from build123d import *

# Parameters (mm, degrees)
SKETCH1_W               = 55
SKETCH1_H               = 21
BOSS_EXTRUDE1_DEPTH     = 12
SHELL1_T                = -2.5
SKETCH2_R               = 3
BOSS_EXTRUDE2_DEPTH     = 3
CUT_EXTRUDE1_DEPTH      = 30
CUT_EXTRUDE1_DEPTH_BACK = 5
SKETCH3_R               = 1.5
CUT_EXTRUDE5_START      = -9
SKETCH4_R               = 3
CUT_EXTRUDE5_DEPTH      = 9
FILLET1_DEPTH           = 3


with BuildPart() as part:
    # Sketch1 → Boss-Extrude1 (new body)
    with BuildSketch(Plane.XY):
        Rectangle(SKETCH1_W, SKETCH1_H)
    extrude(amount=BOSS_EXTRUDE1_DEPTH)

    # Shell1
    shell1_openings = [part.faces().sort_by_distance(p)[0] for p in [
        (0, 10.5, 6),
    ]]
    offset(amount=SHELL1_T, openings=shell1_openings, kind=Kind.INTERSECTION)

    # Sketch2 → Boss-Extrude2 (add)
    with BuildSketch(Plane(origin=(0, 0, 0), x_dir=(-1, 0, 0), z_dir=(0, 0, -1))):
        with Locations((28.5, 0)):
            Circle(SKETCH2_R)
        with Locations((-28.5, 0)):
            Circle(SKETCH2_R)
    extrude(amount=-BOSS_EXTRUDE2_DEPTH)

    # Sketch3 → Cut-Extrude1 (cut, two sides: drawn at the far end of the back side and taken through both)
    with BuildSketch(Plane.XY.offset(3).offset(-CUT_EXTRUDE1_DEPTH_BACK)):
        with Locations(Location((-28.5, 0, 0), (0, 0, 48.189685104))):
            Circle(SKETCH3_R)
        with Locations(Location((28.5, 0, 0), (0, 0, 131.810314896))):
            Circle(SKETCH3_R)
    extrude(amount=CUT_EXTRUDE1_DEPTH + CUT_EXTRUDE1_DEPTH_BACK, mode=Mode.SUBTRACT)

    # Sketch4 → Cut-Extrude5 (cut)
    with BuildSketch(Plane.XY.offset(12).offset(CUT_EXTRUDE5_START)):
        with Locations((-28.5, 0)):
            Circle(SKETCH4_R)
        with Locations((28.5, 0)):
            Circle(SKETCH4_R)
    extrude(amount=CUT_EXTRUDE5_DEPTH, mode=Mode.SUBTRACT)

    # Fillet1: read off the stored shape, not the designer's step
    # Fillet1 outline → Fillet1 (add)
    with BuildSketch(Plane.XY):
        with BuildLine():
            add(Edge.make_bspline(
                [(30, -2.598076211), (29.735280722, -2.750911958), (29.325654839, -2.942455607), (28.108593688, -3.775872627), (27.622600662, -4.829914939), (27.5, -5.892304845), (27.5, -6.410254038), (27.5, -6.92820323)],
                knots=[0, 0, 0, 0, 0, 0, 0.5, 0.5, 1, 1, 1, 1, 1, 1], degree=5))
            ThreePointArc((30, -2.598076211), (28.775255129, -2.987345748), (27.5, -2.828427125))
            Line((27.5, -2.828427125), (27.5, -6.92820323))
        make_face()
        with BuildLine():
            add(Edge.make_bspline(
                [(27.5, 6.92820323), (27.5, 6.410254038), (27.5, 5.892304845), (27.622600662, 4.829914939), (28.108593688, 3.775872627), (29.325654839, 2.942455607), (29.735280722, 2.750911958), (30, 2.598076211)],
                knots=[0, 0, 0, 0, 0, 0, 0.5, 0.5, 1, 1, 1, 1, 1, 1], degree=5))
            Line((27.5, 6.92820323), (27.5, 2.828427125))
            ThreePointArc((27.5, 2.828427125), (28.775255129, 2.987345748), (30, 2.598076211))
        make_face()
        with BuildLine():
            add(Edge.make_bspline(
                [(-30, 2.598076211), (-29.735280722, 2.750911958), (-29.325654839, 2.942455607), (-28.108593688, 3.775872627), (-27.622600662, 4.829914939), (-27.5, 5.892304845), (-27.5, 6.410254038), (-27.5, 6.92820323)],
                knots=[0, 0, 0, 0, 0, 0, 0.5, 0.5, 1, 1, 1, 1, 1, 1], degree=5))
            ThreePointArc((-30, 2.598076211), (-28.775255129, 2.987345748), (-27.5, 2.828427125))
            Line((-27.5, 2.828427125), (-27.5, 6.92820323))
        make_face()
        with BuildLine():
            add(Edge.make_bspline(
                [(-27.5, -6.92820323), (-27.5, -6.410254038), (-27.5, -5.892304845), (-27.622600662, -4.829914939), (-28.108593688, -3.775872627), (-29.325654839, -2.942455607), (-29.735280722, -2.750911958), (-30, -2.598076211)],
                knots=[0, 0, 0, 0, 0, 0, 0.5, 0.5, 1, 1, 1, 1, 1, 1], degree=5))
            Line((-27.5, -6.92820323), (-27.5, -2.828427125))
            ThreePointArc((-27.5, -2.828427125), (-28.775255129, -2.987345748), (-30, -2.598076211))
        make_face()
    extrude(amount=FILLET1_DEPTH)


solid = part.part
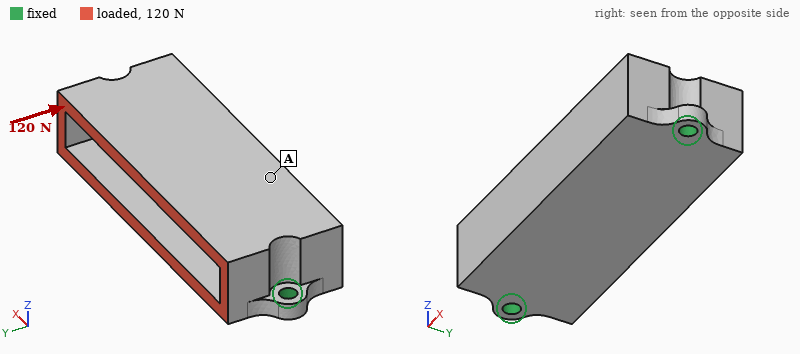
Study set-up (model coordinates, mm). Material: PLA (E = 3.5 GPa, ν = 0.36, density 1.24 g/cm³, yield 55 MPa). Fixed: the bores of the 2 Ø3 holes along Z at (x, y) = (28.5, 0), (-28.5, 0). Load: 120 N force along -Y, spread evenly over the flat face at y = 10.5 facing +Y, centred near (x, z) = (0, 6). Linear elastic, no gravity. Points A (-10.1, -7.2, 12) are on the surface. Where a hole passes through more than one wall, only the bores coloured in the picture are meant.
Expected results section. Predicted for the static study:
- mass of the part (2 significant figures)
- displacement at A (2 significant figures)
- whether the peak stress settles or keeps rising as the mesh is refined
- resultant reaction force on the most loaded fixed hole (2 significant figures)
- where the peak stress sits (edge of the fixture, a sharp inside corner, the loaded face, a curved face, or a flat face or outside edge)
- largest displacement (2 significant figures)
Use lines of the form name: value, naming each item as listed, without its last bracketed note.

mass of the part: 9.1 g
displacement at A: 0.10 mm
whether the peak stress settles or keeps rising as the mesh is refined: keeps rising
resultant reaction force on the most loaded fixed hole: 60 N
where the peak stress sits: edge of the fixture
largest displacement: 0.12 mm
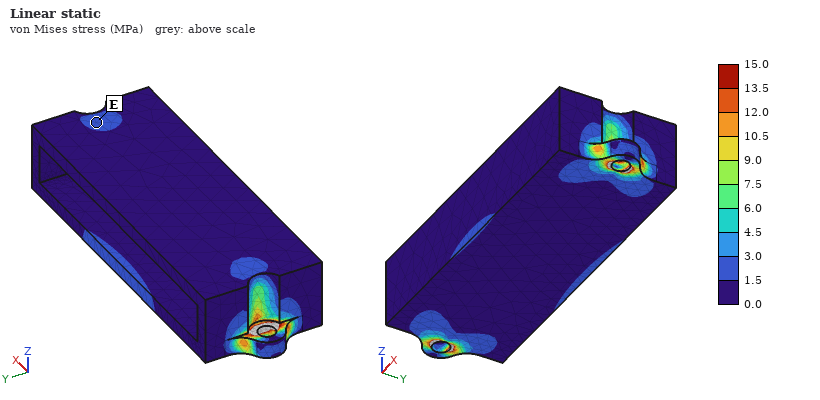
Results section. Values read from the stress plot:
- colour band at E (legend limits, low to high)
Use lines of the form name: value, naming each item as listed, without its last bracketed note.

colour band at E: 1.5 to 3.0 MPa
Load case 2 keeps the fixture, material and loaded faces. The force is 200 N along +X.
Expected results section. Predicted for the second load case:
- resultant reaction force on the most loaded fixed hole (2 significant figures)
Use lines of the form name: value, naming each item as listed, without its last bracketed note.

resultant reaction force on the most loaded fixed hole: 110 N
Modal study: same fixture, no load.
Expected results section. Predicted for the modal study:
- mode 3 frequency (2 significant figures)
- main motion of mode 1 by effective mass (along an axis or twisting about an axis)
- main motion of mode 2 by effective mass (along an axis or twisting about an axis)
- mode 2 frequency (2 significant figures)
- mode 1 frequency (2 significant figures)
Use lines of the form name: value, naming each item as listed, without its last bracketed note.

mode 3 frequency: 2300 Hz
main motion of mode 1 by effective mass: along Y
main motion of mode 2 by effective mass: along Z
mode 2 frequency: 2000 Hz
mode 1 frequency: 1600 Hz
